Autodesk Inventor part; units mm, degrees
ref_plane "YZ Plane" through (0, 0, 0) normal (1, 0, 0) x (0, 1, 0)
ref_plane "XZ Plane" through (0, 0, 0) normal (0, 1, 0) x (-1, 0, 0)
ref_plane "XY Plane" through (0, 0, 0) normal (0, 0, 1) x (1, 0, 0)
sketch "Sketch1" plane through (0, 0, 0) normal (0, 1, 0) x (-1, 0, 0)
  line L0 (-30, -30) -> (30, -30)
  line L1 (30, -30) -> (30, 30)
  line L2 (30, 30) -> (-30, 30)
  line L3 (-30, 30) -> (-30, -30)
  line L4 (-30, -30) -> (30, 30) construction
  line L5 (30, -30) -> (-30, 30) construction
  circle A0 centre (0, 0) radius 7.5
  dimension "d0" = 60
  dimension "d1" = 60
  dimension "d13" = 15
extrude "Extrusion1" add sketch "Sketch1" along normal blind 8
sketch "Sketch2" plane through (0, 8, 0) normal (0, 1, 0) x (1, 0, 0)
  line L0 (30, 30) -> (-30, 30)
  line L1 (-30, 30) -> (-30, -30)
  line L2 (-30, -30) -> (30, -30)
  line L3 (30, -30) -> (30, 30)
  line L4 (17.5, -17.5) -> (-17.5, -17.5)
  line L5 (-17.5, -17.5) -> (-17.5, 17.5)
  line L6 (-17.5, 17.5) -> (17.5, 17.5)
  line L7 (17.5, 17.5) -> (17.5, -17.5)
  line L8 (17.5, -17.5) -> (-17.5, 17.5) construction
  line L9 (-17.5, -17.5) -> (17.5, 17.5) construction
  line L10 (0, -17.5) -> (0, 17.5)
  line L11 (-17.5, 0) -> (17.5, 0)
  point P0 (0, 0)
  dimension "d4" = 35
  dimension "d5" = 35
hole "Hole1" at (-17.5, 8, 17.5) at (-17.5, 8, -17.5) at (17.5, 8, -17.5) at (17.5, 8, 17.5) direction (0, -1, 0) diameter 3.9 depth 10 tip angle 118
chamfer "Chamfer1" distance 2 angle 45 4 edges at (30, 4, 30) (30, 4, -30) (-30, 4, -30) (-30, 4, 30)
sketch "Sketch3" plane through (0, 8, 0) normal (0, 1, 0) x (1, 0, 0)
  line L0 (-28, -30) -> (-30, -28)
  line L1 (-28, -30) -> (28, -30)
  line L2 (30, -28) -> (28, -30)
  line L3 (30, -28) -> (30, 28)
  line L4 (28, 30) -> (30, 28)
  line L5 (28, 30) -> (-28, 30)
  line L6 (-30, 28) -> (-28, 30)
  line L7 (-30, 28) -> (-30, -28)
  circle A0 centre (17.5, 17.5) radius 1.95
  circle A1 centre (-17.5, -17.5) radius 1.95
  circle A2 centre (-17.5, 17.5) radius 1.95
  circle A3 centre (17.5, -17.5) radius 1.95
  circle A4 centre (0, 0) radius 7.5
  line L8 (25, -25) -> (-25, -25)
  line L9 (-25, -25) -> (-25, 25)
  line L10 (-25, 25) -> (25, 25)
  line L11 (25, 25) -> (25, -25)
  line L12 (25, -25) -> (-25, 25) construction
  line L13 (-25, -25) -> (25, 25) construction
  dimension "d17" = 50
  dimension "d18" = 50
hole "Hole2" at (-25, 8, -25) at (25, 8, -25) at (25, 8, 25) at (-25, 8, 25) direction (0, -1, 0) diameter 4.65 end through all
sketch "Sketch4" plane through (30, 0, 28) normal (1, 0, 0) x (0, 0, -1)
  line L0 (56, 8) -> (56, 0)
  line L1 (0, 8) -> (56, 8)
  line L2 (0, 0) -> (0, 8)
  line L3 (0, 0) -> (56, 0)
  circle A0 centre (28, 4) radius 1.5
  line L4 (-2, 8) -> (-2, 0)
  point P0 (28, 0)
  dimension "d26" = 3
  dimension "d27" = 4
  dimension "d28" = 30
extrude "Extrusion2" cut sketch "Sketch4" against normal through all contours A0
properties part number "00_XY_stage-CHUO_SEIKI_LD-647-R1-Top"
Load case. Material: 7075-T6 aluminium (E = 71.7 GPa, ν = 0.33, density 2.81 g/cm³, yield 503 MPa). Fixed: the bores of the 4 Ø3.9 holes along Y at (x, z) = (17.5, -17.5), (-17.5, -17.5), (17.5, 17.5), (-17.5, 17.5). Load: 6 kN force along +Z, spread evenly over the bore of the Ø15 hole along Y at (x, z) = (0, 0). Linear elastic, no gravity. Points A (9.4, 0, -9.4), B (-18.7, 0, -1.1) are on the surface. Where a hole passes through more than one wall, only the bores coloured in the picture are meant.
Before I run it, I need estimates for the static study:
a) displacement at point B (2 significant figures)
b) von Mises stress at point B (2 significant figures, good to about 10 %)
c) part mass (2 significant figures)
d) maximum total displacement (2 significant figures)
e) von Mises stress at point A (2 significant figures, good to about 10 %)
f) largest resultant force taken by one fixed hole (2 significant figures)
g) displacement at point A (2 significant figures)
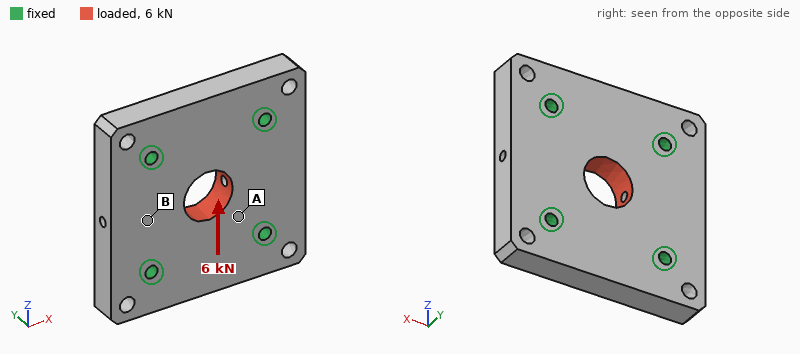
1.2 µm
6.5 MPa
73 g
5.5 µm
15 MPa
1.6 kN
2.9 µm
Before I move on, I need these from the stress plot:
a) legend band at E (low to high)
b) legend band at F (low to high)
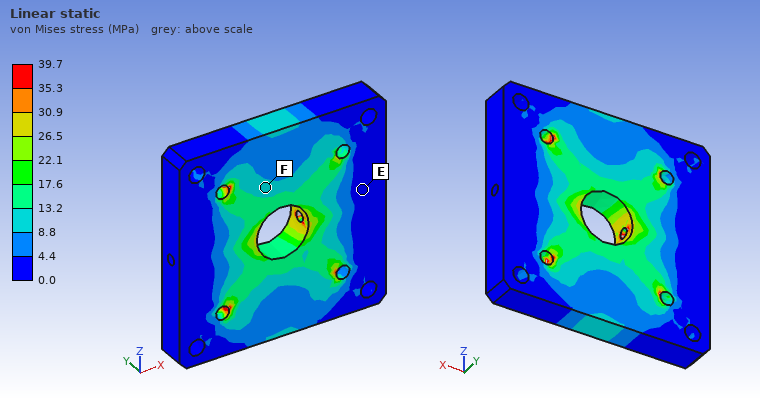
0.0 to 4.4 MPa
8.8 to 13.2 MPa
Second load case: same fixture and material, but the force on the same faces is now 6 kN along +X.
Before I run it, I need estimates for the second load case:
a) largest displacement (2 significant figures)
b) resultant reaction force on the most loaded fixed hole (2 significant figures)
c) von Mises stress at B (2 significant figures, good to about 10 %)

5.4 µm
1.6 kN
6.0 MPa
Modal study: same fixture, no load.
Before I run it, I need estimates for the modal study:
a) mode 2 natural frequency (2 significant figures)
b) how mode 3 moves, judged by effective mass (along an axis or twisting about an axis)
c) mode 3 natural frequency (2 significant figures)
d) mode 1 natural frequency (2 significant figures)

21 kHz
twisting about X
21 kHz
20 kHz
